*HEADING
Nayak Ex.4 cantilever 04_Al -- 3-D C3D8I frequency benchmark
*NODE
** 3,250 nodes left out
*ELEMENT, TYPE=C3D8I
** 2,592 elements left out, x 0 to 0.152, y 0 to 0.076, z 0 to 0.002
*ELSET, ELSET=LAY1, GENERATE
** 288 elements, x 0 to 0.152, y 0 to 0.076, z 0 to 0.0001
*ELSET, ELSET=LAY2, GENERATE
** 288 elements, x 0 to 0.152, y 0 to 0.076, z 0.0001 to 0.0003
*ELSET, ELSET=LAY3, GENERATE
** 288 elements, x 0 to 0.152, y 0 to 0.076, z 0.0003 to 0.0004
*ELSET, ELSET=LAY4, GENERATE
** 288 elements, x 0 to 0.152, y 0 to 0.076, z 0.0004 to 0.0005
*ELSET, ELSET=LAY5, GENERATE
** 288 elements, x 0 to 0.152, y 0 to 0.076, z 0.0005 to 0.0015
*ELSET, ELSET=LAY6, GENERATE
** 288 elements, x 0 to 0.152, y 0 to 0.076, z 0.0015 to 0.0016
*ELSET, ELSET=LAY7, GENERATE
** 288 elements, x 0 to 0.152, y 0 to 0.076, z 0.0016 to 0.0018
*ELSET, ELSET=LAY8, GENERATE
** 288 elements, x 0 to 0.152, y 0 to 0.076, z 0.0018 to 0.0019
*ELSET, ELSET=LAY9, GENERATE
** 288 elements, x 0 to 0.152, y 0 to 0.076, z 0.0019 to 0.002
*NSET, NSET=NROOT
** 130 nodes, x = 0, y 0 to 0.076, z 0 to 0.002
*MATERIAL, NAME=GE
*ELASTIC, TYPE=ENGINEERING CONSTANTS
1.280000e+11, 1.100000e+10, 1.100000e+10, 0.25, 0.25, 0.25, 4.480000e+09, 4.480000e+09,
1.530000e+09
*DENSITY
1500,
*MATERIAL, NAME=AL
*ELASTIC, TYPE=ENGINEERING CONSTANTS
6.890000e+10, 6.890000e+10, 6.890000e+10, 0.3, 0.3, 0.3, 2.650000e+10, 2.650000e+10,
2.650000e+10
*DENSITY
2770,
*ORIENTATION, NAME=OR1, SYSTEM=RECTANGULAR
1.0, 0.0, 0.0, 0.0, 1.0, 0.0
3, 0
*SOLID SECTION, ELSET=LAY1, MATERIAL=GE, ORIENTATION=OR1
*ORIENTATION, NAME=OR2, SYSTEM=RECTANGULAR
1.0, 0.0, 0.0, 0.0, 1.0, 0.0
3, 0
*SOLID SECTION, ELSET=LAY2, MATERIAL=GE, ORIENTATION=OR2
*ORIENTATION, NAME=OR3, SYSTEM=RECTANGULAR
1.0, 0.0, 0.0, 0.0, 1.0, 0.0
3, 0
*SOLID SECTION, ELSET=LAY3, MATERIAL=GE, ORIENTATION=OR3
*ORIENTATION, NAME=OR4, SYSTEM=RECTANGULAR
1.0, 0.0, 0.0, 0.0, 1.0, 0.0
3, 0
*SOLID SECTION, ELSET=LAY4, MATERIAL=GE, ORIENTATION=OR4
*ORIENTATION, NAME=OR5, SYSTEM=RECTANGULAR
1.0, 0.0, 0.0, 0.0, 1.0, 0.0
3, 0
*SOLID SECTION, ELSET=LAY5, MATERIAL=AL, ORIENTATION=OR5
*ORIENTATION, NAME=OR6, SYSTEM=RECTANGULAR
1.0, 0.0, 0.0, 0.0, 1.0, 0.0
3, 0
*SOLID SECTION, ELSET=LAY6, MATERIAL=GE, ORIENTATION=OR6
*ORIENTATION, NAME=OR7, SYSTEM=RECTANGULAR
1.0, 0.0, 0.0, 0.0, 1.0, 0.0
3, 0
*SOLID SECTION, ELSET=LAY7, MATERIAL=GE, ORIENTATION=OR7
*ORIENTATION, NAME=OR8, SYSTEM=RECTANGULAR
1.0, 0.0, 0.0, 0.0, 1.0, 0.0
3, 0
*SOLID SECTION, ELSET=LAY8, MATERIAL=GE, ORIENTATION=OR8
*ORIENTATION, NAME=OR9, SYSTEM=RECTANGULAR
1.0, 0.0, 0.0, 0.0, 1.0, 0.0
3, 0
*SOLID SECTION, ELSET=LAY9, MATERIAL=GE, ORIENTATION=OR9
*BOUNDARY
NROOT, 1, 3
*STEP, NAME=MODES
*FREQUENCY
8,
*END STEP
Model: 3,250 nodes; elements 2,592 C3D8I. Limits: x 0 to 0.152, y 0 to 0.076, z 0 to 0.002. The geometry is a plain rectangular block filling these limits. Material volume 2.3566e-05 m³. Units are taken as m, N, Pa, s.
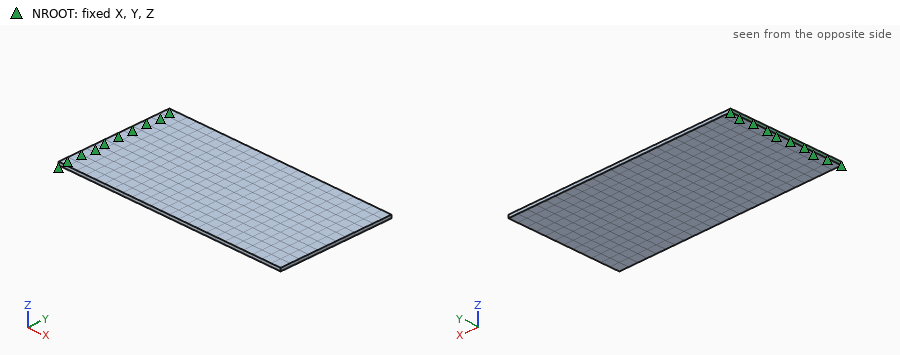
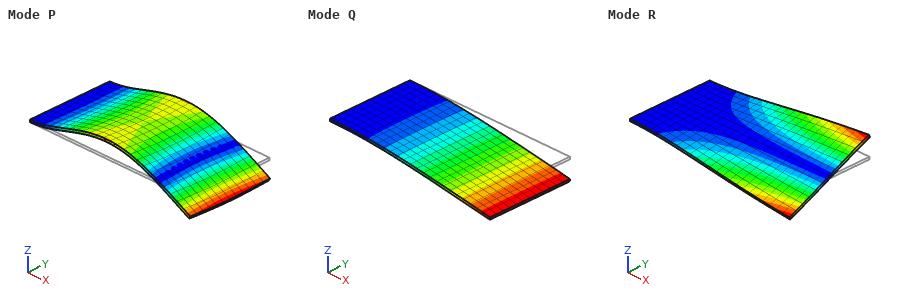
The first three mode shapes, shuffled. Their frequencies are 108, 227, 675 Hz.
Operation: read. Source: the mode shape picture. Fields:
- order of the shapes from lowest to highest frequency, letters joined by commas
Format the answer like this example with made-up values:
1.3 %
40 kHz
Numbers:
Q, R, P
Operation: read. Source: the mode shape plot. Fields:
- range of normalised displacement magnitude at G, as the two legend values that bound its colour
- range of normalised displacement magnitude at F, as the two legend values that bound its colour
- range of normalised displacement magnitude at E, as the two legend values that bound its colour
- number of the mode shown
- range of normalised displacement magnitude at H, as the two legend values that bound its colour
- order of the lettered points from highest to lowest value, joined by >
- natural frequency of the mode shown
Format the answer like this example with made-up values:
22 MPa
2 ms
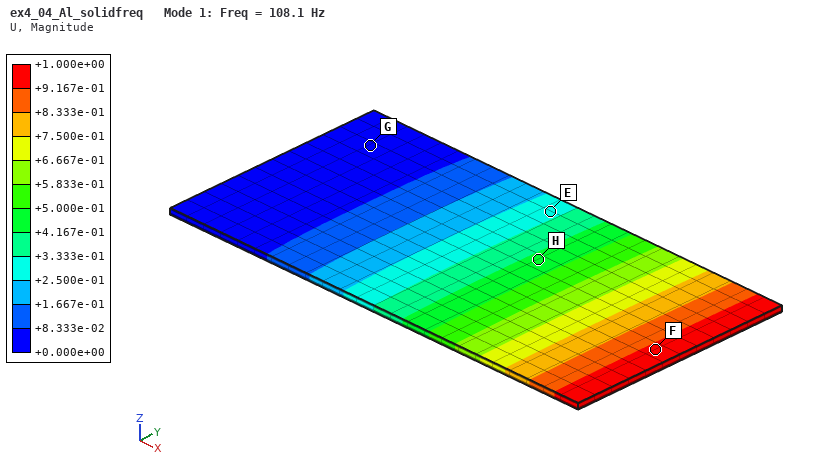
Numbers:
+0.000e+00 to +8.333e-02
+9.167e-01 to +1.000e+00
+2.500e-01 to +3.333e-01
1
+4.167e-01 to +5.000e-01
F > H > E > G
108.1 Hz
